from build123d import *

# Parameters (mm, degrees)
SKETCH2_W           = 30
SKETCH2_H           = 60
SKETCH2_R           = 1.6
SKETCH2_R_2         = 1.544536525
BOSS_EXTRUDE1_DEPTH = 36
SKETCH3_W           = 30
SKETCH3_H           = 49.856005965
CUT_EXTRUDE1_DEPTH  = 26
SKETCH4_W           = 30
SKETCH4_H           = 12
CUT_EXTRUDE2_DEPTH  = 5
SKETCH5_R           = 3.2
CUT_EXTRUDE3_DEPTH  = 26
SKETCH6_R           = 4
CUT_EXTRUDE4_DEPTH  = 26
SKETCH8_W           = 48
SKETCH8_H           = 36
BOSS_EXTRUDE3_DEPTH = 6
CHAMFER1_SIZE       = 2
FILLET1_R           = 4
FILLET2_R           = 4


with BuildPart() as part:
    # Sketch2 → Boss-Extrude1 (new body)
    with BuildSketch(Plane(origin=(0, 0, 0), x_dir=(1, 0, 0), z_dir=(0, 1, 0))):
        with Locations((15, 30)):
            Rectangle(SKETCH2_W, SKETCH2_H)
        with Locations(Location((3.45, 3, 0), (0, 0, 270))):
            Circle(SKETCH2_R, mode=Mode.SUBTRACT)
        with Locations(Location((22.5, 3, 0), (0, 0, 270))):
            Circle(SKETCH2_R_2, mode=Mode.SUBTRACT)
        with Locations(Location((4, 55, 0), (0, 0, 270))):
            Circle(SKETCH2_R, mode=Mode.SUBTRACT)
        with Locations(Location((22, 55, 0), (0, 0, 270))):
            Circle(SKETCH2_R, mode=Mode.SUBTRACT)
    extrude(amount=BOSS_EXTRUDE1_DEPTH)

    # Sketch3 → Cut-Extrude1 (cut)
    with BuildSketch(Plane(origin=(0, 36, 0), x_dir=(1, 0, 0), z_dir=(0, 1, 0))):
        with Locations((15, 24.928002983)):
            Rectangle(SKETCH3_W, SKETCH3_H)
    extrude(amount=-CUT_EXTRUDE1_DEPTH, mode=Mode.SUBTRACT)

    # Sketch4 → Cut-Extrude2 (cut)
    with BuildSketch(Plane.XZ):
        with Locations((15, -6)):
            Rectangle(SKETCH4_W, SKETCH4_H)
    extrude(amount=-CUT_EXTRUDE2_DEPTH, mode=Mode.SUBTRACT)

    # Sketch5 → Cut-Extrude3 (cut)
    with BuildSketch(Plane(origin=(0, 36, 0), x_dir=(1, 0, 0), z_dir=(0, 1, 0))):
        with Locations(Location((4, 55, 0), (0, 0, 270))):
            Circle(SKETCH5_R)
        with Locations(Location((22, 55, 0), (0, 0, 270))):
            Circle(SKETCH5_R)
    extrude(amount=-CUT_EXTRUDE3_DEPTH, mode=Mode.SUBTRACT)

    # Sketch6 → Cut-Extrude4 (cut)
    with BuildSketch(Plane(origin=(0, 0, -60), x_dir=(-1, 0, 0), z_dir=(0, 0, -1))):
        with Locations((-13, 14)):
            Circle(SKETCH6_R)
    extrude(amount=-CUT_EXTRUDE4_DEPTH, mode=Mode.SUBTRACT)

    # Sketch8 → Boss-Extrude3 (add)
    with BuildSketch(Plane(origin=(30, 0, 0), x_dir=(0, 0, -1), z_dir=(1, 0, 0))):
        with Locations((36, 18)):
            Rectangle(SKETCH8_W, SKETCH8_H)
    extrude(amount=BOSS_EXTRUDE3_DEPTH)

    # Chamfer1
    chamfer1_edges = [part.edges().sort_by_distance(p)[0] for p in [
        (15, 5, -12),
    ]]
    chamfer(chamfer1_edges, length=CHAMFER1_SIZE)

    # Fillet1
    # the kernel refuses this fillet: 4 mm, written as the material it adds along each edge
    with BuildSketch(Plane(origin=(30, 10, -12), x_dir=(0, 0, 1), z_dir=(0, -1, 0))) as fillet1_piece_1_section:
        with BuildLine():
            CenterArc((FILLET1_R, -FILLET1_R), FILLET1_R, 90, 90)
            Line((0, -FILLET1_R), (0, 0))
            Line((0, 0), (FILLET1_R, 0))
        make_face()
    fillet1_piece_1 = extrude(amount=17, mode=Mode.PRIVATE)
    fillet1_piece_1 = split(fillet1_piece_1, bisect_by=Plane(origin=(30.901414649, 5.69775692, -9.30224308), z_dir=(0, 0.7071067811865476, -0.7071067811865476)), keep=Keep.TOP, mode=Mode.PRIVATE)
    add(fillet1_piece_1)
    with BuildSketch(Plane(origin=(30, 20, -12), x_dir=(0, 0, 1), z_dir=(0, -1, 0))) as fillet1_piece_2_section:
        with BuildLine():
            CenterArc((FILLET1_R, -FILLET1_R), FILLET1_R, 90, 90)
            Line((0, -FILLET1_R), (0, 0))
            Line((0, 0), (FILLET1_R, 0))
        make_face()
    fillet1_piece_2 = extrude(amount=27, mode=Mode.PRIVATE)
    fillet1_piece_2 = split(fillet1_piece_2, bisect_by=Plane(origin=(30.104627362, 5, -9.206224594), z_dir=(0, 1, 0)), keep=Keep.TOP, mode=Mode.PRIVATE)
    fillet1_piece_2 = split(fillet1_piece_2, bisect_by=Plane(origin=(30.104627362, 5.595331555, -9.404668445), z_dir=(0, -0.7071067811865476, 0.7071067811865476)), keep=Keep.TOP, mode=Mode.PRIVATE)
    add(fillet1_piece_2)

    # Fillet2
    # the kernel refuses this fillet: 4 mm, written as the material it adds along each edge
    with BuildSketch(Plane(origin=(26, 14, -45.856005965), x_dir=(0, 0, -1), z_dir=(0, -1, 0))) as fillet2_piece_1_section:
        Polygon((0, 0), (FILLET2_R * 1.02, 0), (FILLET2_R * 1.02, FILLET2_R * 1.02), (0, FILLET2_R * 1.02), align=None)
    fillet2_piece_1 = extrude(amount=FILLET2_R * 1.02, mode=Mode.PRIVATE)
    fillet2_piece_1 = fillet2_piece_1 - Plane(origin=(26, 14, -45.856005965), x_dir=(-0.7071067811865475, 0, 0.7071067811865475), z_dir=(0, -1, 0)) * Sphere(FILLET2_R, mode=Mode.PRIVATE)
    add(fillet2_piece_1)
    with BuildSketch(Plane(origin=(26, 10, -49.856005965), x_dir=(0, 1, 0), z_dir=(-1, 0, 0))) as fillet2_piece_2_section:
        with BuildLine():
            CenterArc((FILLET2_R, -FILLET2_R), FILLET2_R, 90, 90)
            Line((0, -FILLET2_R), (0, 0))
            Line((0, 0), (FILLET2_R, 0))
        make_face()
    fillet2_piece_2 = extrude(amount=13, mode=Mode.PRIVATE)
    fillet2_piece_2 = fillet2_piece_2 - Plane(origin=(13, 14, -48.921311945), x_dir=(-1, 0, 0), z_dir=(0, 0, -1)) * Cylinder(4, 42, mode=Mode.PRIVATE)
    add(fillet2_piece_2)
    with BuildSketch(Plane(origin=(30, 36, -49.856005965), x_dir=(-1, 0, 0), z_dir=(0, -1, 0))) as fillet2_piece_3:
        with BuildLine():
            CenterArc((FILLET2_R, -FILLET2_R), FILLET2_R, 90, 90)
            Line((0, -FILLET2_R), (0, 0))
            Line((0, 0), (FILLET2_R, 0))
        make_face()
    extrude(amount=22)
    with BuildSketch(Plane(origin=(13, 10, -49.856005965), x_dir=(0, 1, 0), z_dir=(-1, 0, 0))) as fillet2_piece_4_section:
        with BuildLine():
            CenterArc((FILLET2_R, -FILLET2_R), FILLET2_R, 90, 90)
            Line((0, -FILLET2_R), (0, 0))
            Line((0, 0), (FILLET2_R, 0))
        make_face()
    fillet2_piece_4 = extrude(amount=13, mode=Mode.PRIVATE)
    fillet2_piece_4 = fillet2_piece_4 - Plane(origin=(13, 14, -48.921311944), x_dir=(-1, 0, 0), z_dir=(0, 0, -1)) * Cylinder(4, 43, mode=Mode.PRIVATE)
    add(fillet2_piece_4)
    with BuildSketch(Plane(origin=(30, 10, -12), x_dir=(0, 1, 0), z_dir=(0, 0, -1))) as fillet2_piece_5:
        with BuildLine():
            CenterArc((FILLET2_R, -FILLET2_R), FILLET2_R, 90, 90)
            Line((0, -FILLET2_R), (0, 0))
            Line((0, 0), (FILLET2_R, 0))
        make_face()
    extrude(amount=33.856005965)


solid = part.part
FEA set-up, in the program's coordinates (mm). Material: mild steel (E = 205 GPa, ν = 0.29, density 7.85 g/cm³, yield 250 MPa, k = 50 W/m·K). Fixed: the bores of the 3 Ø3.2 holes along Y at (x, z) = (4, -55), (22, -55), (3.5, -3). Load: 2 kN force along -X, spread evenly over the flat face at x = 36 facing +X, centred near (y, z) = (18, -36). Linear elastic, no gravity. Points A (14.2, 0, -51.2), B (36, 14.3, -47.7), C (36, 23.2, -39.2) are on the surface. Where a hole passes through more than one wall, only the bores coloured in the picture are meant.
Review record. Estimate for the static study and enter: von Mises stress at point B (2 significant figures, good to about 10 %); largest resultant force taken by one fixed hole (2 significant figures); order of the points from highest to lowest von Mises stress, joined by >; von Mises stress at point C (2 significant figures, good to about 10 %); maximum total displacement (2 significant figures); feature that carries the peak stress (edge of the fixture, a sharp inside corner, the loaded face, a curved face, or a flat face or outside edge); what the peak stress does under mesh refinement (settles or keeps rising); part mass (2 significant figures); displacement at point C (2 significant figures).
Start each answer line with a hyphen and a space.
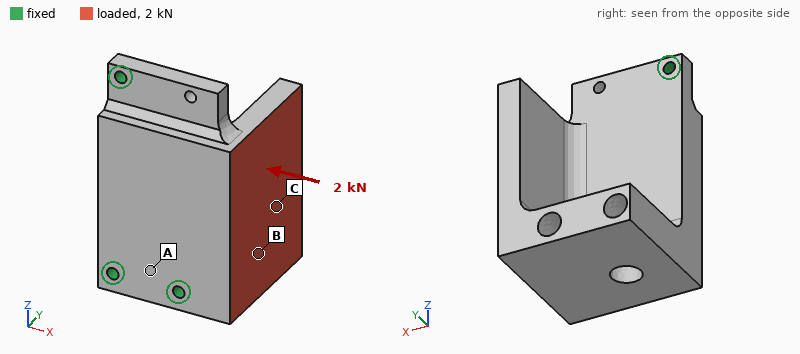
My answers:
- 12 MPa
- 1.2 kN
- C > B > A
- 19 MPa
- 24 µm
- edge of the fixture
- keeps rising
- 250 g
- 7.3 µm
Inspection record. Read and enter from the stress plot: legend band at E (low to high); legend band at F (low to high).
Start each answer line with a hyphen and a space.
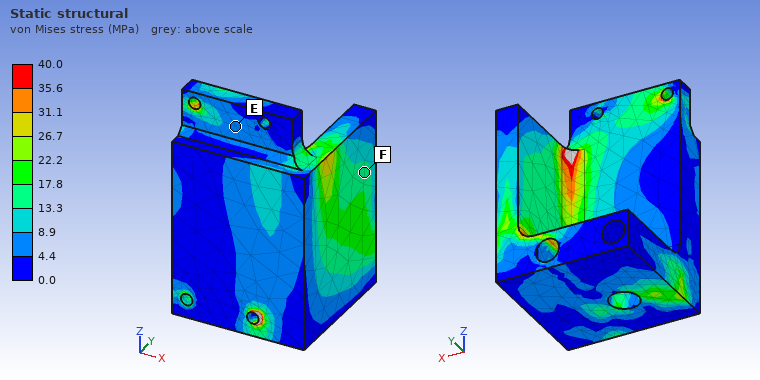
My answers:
- 4.4 to 8.9 MPa
- 13.3 to 17.8 MPa
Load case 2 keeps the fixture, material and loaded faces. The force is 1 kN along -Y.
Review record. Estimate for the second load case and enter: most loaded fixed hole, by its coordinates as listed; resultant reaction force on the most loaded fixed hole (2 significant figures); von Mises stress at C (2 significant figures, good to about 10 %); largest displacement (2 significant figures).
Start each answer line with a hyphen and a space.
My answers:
- (22, -55)
- 1.3 kN
- 6.7 MPa
- 15 µm
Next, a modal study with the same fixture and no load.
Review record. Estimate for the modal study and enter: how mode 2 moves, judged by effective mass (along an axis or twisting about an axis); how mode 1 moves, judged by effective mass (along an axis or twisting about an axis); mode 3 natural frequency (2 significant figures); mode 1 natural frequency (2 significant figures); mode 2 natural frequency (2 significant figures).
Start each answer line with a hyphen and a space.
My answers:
- along X
- along Y
- 11 kHz
- 4600 Hz
- 7600 Hz
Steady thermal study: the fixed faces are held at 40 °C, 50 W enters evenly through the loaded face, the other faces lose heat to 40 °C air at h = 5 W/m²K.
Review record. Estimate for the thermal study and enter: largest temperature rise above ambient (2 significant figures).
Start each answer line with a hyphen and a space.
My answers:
- 71 K
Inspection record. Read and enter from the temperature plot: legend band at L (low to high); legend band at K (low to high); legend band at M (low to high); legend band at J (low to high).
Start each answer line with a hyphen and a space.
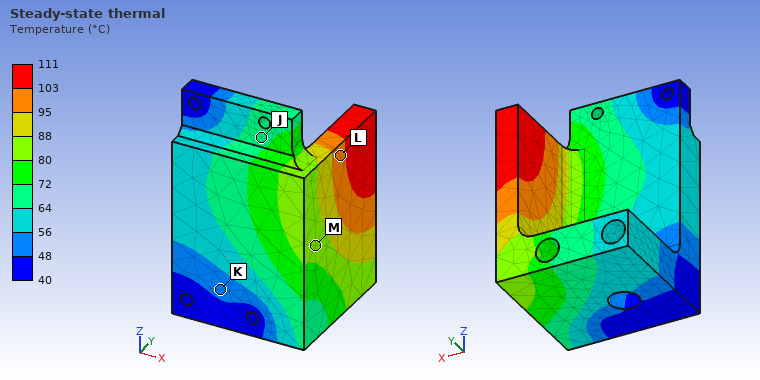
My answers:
- 95 to 103 °C
- 48 to 56 °C
- 80 to 88 °C
- 64 to 72 °C
